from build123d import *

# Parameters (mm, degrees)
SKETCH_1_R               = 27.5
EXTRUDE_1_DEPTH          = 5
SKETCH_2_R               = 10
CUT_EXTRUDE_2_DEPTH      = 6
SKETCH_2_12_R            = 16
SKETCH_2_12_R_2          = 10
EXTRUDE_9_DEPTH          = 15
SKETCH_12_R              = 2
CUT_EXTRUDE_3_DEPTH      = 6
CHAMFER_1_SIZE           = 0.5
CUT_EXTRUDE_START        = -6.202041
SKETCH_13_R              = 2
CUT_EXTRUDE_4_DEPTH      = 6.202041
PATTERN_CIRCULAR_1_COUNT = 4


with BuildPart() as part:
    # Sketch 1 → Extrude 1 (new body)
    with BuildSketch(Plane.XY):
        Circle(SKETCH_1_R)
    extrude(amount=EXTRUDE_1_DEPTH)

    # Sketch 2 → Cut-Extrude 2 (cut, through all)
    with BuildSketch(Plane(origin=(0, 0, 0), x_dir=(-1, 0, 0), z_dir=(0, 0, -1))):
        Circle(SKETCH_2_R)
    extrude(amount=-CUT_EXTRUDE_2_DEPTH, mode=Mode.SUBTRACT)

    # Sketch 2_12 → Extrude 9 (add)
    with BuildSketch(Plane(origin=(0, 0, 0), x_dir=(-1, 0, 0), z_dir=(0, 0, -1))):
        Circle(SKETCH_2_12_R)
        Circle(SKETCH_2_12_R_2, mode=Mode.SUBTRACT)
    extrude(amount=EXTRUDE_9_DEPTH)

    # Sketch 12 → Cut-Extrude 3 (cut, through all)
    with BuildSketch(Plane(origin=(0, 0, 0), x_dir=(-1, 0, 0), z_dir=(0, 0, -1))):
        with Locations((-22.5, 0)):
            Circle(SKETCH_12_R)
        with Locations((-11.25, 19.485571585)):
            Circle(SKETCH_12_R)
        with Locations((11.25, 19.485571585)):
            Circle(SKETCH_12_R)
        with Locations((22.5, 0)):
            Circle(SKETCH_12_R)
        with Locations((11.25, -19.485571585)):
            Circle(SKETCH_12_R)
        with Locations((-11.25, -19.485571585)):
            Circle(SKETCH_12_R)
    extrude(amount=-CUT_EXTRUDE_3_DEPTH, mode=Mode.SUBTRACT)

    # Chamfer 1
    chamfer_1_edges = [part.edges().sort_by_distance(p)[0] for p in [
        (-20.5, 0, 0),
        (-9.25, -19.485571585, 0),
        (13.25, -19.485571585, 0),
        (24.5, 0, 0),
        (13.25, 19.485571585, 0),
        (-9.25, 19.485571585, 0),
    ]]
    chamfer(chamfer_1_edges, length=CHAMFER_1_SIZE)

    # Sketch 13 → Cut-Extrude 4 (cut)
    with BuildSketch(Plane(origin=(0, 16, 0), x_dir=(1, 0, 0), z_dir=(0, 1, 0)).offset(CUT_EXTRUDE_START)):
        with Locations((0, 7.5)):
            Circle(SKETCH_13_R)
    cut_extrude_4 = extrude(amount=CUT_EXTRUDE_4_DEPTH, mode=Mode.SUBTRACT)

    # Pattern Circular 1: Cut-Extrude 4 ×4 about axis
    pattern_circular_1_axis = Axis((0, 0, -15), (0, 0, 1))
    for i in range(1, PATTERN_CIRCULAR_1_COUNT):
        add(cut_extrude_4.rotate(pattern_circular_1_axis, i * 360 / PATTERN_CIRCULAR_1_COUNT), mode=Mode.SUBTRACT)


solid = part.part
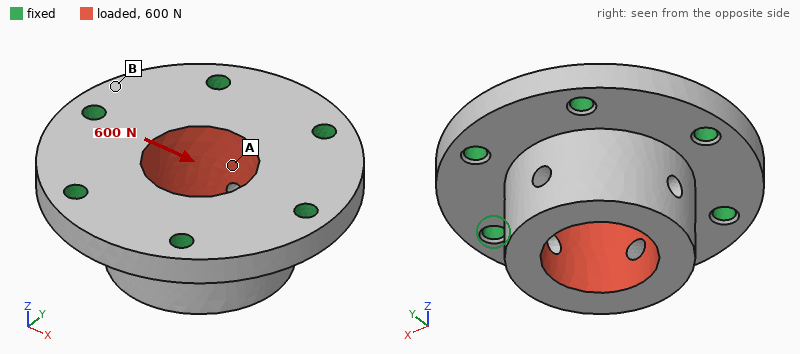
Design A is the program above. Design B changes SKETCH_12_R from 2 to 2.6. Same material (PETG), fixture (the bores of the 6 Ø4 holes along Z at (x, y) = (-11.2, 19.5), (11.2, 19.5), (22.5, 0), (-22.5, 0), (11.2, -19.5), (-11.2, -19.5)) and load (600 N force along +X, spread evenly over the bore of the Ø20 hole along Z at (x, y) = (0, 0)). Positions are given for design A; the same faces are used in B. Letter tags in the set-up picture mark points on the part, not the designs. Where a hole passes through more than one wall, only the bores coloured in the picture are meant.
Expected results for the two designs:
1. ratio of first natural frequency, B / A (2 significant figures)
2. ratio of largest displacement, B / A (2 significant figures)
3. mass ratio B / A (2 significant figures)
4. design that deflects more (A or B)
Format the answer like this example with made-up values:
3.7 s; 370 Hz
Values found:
1.1; 0.91; 0.98; A
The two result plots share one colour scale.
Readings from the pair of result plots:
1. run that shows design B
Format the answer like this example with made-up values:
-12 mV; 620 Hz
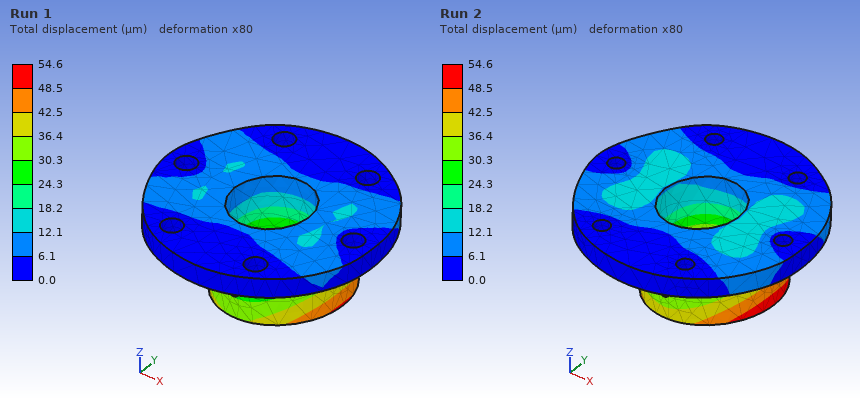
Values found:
Run 1
